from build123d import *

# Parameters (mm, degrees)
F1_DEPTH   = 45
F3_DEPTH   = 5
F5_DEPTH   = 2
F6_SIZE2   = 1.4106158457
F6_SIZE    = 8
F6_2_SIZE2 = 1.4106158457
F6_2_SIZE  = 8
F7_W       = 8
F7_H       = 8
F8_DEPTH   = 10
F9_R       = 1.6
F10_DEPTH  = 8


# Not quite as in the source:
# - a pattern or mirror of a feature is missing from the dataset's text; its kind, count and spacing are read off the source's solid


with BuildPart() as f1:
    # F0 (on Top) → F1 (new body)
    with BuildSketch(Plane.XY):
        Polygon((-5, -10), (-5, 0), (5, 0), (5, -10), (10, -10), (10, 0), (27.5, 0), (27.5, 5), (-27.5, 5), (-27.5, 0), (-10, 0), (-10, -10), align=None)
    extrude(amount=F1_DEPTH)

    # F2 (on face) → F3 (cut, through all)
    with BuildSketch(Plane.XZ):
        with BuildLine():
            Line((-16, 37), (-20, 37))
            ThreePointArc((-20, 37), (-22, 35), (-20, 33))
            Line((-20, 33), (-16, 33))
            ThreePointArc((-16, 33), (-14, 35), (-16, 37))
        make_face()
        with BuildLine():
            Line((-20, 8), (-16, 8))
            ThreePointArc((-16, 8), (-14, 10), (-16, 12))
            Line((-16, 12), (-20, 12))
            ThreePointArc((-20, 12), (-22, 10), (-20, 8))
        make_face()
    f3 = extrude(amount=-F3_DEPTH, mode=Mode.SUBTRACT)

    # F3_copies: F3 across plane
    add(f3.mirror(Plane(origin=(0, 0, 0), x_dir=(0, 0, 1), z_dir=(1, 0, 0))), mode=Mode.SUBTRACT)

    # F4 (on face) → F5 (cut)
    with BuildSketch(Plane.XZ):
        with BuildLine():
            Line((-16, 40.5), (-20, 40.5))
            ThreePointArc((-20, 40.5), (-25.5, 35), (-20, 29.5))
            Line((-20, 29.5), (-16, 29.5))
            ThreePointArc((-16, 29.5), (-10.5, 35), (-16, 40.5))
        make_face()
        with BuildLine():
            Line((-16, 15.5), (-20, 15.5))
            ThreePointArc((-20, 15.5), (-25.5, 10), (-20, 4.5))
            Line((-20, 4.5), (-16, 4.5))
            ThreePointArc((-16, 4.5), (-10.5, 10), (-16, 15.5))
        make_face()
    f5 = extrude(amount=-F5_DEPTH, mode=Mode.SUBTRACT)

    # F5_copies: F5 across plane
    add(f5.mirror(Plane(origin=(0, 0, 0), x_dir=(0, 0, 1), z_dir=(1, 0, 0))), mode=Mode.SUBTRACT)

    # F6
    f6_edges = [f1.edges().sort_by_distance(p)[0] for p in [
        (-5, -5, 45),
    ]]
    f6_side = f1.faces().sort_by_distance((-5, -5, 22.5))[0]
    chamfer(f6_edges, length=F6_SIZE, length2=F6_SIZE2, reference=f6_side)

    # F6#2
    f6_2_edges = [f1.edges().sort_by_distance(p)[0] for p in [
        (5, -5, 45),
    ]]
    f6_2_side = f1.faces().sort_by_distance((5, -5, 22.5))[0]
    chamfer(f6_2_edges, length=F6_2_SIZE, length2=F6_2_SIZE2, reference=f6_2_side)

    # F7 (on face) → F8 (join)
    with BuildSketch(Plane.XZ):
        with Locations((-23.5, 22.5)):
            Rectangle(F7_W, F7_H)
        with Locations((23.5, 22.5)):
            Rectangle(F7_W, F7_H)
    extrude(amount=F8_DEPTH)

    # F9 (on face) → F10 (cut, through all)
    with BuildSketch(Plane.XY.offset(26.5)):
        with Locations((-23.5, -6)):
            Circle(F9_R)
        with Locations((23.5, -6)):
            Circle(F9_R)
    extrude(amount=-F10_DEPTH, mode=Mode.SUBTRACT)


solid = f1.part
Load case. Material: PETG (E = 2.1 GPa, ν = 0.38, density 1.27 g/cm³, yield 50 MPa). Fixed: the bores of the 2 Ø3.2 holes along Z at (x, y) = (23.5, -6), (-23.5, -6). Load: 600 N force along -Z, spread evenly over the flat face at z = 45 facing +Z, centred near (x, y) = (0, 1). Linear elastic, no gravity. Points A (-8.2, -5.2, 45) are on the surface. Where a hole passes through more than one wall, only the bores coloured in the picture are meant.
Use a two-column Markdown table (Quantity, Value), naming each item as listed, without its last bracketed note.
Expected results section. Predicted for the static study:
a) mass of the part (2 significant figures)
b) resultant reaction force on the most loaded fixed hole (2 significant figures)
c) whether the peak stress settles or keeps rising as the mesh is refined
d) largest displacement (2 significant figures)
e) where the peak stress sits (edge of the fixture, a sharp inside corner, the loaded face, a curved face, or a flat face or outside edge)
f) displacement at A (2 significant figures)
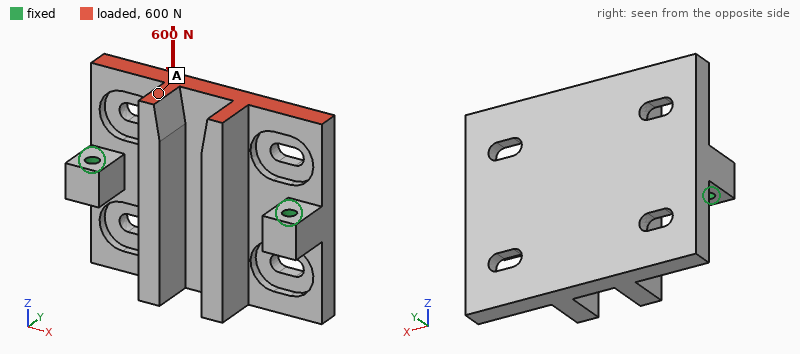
| Quantity | Value |
|---|---|
| mass of the part | 21 g |
| resultant reaction force on the most loaded fixed hole | 300 N |
| whether the peak stress settles or keeps rising as the mesh is refined | keeps rising |
| largest displacement | 0.20 mm |
| where the peak stress sits | edge of the fixture |
| displacement at A | 0.15 mm |
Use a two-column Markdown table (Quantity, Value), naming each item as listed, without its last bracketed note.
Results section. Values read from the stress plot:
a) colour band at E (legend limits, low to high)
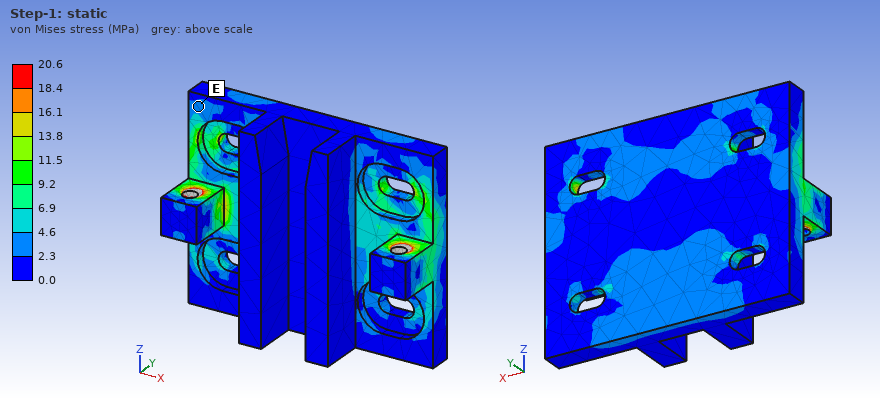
| Quantity | Value |
|---|---|
| colour band at E | 2.3 to 4.6 MPa |
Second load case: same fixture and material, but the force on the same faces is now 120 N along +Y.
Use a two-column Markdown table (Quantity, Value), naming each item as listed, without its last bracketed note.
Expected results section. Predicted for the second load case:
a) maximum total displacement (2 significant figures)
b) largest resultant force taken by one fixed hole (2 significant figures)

| Quantity | Value |
|---|---|
| maximum total displacement | 0.85 mm |
| largest resultant force taken by one fixed hole | 72 N |
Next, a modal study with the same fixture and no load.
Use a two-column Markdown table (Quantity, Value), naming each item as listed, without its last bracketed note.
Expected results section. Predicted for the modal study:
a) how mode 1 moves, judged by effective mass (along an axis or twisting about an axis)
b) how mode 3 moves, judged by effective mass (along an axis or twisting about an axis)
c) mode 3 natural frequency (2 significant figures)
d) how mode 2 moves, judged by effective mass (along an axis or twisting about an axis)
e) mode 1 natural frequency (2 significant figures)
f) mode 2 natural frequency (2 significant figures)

| Quantity | Value |
|---|---|
| how mode 1 moves, judged by effective mass | twisting about X |
| how mode 3 moves, judged by effective mass | along X |
| mode 3 natural frequency | 2000 Hz |
| how mode 2 moves, judged by effective mass | along Y |
| mode 1 natural frequency | 820 Hz |
| mode 2 natural frequency | 1500 Hz |
